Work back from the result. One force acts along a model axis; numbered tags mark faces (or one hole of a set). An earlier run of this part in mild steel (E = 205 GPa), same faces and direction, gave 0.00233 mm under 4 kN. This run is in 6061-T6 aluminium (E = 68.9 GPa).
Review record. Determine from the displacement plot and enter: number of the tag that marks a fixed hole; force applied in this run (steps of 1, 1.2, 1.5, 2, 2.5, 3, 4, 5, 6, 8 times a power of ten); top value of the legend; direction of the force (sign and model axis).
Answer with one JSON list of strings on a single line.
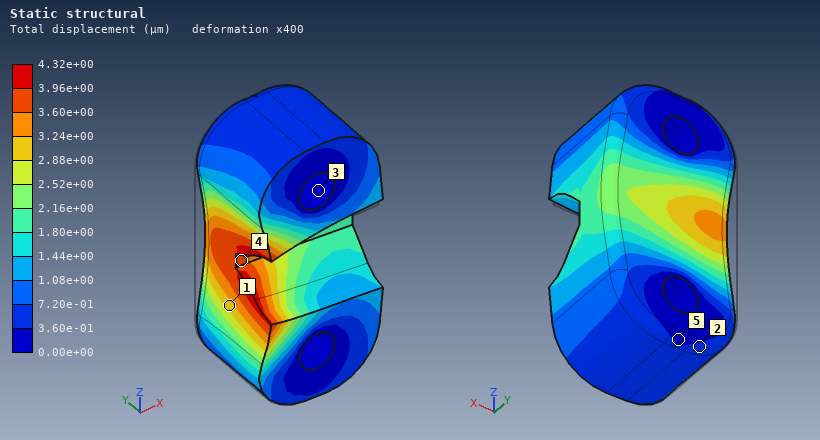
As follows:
["3", "2.5 kN", "4.32e+00 µm", "+X"]
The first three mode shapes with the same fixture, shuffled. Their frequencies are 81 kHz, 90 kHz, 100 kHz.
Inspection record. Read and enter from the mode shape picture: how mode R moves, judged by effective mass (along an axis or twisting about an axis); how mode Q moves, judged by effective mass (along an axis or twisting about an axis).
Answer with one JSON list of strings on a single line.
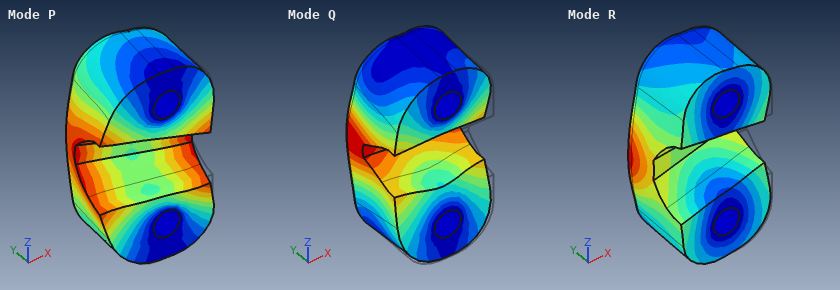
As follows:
["along X", "along Y"]
